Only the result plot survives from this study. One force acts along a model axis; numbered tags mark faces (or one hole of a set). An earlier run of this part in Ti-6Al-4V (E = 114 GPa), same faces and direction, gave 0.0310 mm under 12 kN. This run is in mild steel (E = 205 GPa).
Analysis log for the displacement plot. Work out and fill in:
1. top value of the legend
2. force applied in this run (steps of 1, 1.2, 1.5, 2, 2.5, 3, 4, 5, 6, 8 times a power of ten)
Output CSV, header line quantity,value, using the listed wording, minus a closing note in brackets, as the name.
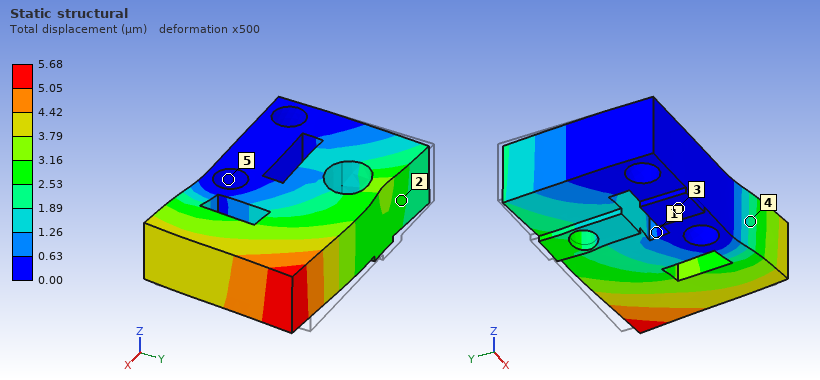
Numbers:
quantity,value
top value of the legend,5.68 µm
force applied in this run,4 kN
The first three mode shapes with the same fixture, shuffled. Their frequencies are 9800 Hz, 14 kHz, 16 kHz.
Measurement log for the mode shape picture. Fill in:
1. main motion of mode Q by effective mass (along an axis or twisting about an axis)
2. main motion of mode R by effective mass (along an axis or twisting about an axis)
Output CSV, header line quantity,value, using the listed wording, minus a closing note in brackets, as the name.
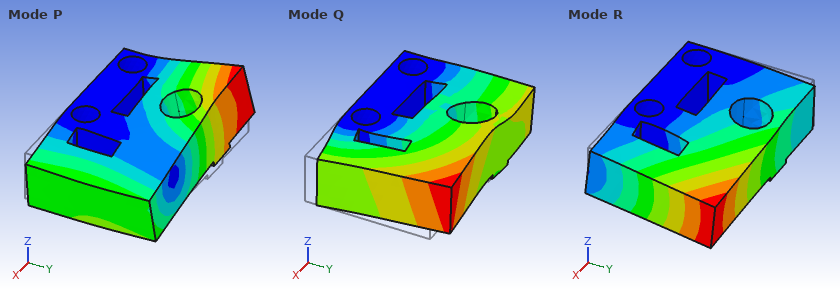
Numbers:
quantity,value
main motion of mode Q by effective mass,along X
main motion of mode R by effective mass,along Z
